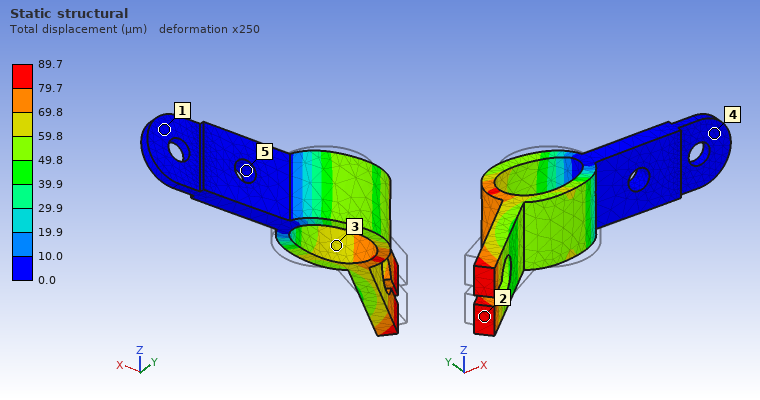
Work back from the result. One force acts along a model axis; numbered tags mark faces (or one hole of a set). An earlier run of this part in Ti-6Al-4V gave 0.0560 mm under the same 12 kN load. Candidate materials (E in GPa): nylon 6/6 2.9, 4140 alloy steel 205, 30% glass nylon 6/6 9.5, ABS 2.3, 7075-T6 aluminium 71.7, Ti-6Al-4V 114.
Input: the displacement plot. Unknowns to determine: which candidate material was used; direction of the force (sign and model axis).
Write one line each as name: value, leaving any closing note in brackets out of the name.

which candidate material was used: 7075-T6 aluminium
direction of the force: -X
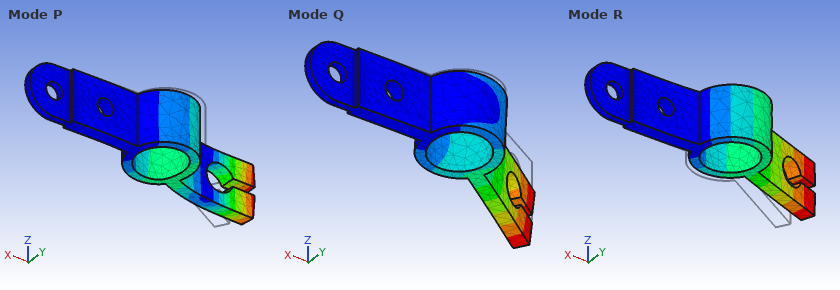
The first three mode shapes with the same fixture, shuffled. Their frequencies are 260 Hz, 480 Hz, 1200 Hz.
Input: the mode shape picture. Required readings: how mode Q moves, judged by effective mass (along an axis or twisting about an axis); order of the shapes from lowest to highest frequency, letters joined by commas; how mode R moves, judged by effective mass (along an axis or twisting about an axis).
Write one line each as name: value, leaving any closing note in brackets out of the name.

how mode Q moves, judged by effective mass: along Z
order of the shapes from lowest to highest frequency, letters joined by commas: R, Q, P
how mode R moves, judged by effective mass: along Y
